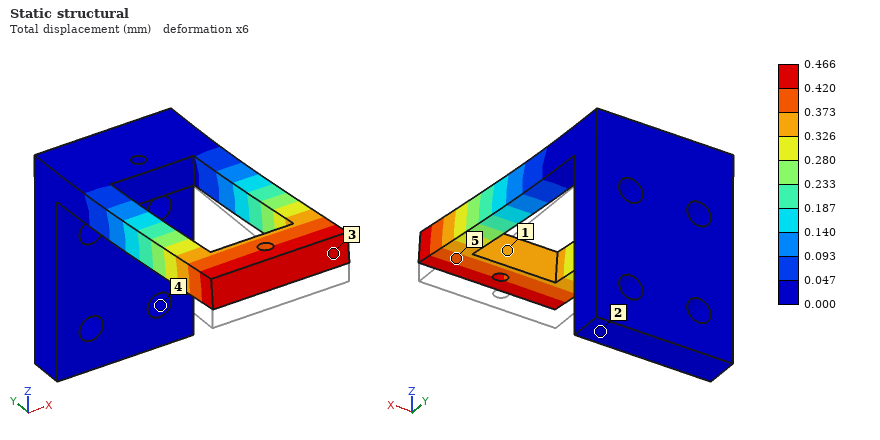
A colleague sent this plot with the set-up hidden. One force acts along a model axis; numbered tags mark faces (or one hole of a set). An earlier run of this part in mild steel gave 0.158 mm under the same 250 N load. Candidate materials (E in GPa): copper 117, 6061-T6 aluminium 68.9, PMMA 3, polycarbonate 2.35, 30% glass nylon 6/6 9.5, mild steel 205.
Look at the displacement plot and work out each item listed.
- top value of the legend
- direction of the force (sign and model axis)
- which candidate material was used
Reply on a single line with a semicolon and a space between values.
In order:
0.466 mm; +Z; 6061-T6 aluminium
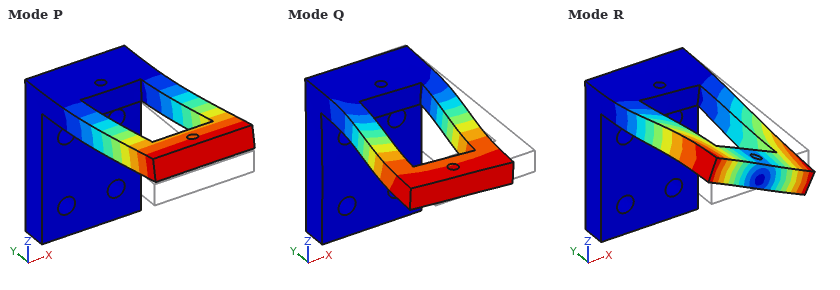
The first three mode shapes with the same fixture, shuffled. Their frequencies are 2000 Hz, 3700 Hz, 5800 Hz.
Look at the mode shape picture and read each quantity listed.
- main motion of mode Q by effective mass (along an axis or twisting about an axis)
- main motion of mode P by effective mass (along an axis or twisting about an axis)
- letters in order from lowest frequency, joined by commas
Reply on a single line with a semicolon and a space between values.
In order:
along X; along Z; P, Q, R
